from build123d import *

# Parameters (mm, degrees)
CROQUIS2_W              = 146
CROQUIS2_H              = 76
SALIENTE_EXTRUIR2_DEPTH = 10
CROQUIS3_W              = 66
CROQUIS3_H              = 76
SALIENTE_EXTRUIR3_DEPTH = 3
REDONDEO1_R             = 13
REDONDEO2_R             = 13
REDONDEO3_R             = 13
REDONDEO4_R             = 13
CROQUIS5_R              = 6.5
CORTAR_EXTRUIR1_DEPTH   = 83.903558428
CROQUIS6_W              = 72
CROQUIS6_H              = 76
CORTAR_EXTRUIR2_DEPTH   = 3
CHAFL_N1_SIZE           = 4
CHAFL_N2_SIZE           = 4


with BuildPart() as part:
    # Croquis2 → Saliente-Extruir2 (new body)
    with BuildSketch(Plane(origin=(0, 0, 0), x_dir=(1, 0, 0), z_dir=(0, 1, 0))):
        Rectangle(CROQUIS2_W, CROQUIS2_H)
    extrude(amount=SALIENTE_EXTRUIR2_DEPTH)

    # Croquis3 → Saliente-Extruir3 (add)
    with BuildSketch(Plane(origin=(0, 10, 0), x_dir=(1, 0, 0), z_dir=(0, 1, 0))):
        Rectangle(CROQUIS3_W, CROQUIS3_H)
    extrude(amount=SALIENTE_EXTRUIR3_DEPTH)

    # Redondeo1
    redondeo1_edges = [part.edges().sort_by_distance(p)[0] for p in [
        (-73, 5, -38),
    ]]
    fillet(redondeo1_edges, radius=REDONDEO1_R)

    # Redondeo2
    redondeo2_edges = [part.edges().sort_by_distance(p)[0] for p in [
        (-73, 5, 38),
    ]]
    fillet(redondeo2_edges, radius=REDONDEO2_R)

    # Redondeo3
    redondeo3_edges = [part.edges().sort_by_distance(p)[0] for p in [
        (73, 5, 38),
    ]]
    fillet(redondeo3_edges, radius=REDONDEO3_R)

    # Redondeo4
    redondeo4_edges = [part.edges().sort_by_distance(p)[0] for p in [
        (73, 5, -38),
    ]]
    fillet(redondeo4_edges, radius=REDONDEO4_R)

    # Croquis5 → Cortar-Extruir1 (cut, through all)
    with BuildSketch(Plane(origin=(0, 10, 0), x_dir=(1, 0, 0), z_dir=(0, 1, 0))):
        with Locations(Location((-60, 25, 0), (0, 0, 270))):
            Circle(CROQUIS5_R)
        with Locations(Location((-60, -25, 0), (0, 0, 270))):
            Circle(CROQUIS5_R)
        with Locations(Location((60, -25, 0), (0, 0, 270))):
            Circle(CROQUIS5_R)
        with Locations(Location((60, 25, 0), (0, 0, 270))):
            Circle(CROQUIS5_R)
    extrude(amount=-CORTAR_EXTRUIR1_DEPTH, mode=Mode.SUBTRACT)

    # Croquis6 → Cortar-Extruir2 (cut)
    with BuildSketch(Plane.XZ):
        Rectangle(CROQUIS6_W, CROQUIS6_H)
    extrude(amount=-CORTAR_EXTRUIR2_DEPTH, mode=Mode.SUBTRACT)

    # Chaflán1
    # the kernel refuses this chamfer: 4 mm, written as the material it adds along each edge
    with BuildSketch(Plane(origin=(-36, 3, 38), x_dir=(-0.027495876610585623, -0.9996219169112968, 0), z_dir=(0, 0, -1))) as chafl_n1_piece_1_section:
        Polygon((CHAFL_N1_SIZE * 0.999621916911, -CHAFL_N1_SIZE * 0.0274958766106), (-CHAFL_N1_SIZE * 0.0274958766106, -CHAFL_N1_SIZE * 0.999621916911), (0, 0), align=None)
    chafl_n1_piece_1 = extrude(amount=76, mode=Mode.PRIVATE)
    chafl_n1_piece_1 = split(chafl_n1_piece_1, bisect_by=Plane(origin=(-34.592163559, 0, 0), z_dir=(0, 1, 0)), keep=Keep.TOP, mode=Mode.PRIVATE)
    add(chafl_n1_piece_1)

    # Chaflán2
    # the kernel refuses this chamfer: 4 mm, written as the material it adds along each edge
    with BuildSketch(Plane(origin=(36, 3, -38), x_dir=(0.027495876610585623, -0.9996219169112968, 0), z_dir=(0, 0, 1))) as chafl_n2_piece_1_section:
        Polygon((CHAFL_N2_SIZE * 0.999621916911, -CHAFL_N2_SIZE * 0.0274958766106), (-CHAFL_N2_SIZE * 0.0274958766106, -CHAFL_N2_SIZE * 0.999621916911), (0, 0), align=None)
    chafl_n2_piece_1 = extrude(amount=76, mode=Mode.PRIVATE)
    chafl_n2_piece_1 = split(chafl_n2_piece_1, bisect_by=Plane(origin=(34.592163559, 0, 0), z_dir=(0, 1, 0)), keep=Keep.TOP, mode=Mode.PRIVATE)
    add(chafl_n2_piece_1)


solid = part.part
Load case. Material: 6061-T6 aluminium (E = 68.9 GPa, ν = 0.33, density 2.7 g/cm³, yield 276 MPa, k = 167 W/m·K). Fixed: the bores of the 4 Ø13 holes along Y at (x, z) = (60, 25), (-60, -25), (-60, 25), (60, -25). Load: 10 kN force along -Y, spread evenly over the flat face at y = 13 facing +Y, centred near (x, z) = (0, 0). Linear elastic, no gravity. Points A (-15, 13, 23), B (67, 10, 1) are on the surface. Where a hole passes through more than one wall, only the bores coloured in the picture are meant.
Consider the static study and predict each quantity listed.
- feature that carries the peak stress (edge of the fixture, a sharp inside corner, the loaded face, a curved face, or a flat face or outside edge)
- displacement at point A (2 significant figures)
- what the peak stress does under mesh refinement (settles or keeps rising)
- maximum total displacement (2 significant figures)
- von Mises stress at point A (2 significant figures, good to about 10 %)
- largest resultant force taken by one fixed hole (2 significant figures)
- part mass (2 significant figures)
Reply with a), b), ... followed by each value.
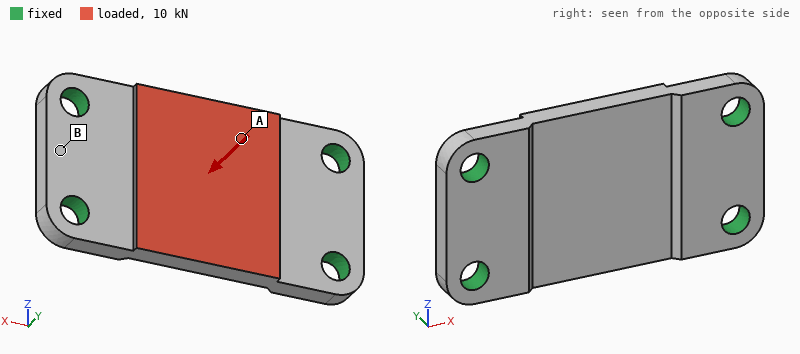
a) edge of the fixture
b) 0.11 mm
c) keeps rising
d) 0.13 mm
e) 46 MPa
f) 4.5 kN
g) 280 g
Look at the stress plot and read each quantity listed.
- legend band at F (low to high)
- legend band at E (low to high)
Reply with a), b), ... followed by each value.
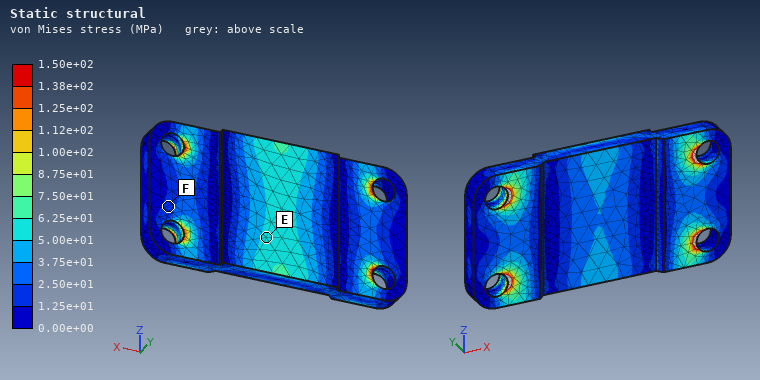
a) 1.25e+01 to 2.50e+01 MPa
b) 5.00e+01 to 6.25e+01 MPa
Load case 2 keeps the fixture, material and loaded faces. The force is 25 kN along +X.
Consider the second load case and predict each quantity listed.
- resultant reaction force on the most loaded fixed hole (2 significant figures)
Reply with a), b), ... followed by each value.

a) 6.4 kN
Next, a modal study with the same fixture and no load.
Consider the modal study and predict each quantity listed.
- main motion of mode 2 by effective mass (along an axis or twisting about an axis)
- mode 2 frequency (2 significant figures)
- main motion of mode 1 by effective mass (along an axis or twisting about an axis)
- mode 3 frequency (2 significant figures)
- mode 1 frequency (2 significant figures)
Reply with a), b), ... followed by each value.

a) twisting about X
b) 5400 Hz
c) along Y
d) 9400 Hz
e) 4100 Hz
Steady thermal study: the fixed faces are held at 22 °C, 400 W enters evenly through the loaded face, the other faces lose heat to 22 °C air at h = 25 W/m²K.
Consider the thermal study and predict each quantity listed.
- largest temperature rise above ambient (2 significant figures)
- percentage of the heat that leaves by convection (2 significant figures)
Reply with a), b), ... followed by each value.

a) 70 K
b) 3.7 %
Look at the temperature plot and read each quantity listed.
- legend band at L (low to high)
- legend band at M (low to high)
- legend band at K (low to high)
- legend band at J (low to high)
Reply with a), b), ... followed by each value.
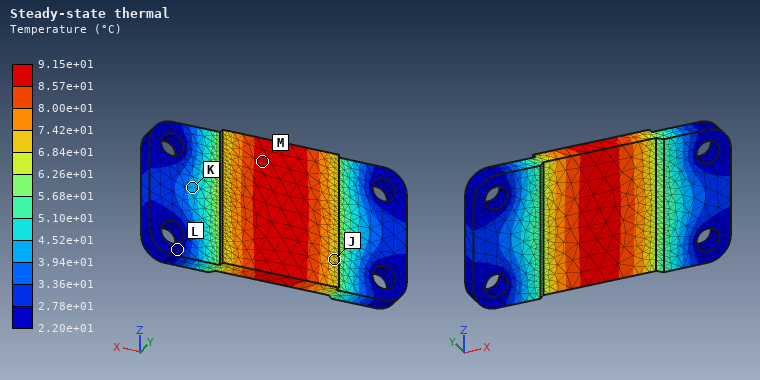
a) 2.20e+01 to 2.78e+01 °C
b) 8.57e+01 to 9.15e+01 °C
c) 3.94e+01 to 4.52e+01 °C
d) 6.84e+01 to 7.42e+01 °C
